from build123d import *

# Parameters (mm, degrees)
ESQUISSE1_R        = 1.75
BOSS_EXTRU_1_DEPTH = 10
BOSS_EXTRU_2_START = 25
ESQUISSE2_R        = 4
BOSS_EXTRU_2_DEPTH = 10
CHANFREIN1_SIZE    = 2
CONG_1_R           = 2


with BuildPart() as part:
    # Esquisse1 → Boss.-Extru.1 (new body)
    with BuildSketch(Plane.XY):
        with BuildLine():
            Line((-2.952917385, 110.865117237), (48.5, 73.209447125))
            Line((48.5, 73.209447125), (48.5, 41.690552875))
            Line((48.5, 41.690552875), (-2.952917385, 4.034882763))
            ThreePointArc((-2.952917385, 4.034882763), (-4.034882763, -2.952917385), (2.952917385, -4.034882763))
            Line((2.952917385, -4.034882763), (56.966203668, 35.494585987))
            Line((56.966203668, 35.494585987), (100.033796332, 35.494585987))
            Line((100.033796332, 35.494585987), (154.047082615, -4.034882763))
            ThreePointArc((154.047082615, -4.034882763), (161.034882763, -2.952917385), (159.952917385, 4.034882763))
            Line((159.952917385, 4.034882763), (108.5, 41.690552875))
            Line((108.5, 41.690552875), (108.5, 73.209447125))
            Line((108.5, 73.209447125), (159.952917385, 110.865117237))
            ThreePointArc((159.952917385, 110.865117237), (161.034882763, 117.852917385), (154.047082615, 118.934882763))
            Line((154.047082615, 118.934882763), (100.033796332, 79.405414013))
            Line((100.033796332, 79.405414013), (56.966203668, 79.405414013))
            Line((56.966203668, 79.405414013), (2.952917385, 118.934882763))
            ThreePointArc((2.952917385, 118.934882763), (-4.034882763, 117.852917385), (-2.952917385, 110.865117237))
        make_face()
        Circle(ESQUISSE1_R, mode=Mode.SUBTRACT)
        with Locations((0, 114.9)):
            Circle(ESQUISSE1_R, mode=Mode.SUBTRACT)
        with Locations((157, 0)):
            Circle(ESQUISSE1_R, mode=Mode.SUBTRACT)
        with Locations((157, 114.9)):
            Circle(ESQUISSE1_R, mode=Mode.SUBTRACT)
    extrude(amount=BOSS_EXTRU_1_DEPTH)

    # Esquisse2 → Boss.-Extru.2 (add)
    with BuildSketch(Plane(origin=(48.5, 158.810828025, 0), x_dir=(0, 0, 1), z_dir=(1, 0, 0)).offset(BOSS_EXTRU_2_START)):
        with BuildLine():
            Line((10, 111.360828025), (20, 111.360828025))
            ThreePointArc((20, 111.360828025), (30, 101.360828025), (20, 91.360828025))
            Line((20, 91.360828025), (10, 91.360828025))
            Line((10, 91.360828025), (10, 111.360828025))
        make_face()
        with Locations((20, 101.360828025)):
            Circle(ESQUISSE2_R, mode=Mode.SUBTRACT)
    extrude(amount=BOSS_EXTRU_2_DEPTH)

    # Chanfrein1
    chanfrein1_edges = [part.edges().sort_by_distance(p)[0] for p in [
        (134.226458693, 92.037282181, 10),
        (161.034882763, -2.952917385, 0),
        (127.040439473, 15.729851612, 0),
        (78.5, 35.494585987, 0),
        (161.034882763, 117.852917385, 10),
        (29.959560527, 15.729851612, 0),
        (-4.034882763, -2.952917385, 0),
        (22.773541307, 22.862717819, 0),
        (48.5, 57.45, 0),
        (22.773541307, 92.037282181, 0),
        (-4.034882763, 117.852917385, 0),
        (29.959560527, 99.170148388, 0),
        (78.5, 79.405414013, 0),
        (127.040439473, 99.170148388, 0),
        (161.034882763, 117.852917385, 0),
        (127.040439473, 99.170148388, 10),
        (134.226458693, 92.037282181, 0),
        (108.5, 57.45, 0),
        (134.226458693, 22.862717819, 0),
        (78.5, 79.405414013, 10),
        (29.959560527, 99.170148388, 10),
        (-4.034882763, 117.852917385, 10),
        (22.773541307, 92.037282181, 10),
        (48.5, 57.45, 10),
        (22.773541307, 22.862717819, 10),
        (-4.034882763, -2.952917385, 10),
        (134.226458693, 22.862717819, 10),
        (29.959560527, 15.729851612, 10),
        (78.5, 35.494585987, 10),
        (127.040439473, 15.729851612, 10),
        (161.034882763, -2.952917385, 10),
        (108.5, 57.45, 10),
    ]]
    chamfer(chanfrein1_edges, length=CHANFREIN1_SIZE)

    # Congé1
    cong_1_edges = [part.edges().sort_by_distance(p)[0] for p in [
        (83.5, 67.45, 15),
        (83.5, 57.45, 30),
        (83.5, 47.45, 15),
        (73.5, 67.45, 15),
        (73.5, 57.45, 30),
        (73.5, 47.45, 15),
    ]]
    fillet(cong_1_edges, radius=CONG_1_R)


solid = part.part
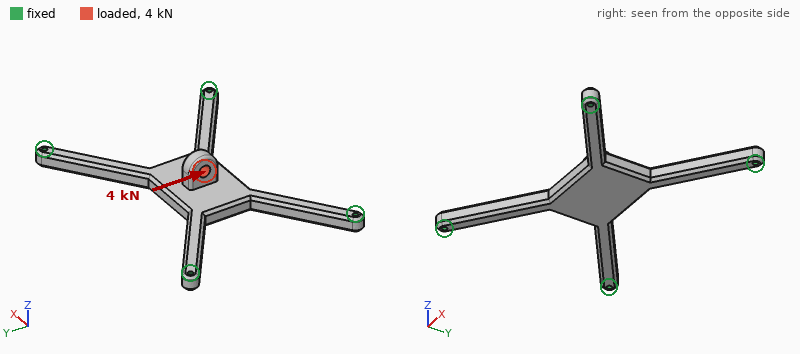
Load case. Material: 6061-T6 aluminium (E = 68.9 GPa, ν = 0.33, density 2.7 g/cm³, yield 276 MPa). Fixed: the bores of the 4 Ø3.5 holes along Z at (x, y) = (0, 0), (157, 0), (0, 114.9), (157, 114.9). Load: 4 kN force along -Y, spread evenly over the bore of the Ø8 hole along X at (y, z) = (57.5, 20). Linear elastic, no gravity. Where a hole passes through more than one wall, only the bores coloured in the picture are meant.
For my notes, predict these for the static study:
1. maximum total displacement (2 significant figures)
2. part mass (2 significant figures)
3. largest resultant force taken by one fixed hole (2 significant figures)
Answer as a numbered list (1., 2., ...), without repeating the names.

1. 0.27 mm
2. 140 g
3. 1.7 kN
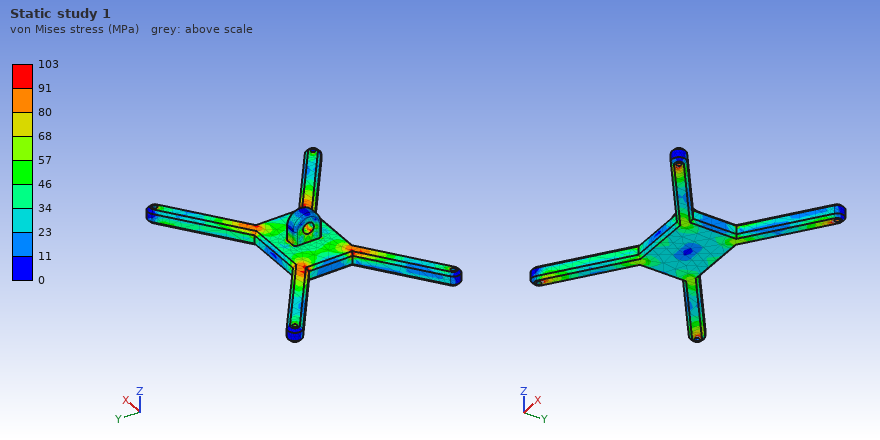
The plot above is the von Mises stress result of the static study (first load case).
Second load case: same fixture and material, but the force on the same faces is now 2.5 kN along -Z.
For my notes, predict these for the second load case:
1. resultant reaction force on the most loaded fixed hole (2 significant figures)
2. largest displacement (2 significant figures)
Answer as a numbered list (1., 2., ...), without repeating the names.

1. 630 N
2. 0.56 mm
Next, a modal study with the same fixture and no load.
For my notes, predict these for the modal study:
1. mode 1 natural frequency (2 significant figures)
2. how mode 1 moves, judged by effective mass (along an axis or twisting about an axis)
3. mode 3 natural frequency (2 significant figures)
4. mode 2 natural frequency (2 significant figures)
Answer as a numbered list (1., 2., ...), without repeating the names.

1. 1200 Hz
2. along Z
3. 3100 Hz
4. 3100 Hz
